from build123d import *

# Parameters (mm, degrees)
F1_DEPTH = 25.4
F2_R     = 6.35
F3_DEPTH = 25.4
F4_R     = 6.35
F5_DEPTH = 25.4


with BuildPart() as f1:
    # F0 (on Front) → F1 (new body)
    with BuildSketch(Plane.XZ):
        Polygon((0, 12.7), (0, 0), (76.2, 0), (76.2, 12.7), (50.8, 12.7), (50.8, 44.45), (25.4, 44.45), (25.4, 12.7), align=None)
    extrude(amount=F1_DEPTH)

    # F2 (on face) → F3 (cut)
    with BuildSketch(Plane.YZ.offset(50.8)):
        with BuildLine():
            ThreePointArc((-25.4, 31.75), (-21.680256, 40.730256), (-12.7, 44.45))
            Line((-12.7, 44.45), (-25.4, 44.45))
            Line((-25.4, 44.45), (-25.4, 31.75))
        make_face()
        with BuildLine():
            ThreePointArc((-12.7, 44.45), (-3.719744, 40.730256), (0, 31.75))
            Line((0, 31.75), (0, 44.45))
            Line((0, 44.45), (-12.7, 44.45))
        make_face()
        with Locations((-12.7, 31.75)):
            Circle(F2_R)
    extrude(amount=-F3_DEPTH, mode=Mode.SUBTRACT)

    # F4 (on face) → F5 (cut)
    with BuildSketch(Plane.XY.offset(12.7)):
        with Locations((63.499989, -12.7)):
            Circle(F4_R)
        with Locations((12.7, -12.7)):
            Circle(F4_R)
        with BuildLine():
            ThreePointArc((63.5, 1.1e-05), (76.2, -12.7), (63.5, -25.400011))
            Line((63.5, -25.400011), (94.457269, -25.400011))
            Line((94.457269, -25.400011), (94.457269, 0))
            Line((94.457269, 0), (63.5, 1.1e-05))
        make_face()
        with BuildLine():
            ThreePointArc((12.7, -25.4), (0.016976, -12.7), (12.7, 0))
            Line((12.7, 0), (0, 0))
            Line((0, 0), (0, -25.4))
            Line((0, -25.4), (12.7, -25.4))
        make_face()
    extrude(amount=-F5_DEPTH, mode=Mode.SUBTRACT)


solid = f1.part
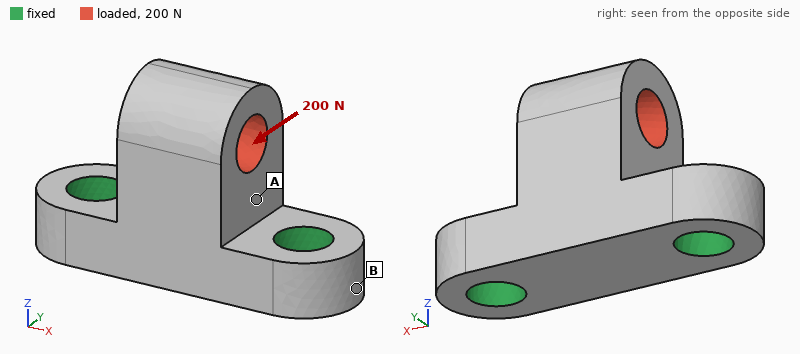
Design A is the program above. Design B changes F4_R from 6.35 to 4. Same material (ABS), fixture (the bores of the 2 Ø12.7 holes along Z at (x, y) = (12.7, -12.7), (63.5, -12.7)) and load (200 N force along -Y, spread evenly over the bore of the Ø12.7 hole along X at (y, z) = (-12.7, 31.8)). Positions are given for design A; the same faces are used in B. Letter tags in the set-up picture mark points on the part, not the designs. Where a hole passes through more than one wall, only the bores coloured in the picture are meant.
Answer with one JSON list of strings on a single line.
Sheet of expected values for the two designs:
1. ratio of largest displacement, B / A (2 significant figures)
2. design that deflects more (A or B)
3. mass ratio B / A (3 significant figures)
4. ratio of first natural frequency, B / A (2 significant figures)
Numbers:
["1.3", "B", "1.06", "0.88"]
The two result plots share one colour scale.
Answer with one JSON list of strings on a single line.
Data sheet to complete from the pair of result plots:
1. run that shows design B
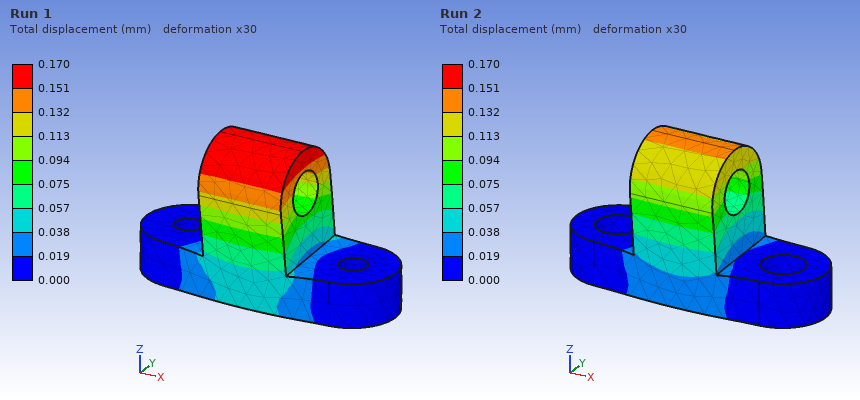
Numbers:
["Run 1"]
